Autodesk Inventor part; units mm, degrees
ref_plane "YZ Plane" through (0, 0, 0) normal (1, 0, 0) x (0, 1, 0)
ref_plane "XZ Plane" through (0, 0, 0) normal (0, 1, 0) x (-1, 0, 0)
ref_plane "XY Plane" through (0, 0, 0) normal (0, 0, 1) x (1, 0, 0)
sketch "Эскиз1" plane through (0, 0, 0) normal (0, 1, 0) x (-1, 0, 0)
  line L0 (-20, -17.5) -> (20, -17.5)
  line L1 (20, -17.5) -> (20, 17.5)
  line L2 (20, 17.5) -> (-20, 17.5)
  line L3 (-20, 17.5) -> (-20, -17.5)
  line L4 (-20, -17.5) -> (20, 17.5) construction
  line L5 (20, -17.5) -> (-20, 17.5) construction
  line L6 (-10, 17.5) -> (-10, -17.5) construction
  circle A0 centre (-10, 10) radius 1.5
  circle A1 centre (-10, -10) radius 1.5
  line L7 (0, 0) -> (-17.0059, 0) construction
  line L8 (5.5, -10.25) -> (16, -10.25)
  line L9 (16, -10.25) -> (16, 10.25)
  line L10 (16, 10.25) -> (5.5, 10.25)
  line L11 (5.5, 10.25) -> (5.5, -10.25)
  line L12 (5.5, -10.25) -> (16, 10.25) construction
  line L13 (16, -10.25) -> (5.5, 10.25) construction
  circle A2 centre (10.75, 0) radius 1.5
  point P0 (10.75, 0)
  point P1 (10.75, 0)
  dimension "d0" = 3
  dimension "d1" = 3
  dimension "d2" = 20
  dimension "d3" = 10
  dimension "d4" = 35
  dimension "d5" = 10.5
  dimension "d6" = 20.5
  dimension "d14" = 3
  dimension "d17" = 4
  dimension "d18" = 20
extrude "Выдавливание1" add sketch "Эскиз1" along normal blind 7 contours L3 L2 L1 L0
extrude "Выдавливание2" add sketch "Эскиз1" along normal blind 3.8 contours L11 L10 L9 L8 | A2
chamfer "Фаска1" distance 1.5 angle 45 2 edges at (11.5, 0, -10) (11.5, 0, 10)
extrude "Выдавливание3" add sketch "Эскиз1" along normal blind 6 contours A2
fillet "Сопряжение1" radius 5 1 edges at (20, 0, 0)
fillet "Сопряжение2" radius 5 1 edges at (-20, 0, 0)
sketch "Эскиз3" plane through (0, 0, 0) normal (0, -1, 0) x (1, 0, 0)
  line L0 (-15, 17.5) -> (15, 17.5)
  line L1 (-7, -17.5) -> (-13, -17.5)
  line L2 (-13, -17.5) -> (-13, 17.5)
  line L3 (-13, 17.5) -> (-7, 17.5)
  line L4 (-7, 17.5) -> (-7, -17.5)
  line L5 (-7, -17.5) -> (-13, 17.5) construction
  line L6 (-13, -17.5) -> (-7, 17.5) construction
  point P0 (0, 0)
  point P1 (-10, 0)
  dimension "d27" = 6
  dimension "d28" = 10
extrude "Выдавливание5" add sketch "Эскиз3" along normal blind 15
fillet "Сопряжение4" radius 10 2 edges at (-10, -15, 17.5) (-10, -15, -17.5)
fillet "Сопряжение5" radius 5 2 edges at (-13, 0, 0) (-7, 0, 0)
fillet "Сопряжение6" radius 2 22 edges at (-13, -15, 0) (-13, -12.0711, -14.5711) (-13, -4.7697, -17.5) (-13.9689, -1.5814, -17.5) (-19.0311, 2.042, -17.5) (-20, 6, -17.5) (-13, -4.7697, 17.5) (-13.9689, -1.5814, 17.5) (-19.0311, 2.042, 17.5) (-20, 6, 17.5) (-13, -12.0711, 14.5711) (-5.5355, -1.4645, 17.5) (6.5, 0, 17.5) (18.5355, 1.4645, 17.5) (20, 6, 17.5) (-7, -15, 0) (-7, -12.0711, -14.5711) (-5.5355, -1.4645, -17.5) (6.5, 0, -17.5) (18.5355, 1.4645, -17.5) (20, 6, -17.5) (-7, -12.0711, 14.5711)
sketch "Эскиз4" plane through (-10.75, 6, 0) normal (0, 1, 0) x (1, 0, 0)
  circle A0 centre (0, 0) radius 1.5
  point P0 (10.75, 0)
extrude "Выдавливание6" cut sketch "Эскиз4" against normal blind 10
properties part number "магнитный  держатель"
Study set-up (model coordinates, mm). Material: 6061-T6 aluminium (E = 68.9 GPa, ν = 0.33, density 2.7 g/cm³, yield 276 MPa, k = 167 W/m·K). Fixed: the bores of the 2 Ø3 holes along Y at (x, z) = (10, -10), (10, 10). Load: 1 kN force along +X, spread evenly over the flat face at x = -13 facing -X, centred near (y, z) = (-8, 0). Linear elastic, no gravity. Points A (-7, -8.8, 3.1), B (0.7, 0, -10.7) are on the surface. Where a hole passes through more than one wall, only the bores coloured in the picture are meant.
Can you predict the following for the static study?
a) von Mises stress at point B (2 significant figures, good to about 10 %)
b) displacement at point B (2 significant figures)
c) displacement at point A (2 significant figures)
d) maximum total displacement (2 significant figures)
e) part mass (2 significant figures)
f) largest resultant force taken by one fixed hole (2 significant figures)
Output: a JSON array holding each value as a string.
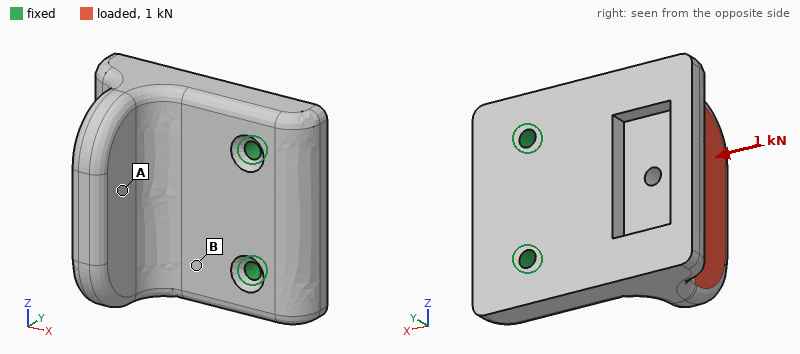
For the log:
["46 MPa", "0.017 mm", "0.066 mm", "0.10 mm", "31 g", "510 N"]
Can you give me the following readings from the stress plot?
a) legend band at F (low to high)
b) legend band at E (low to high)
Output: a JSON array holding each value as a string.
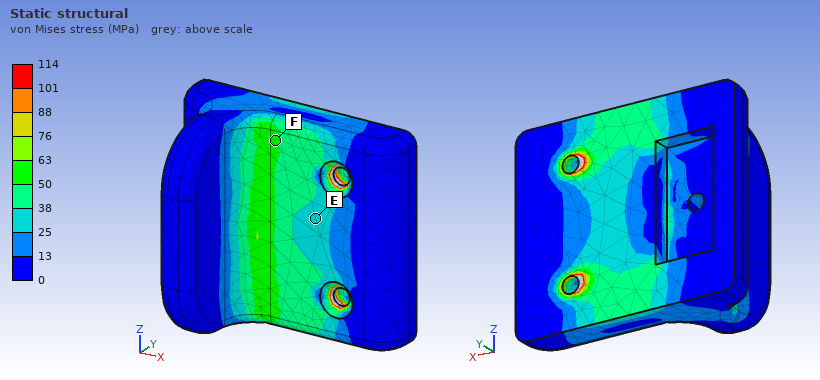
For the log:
["50 to 63 MPa", "25 to 38 MPa"]
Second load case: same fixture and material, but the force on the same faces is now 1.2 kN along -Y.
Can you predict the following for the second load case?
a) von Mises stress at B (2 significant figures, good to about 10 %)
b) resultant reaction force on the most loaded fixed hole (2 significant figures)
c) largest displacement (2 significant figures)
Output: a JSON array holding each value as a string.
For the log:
["57 MPa", "600 N", "0.16 mm"]
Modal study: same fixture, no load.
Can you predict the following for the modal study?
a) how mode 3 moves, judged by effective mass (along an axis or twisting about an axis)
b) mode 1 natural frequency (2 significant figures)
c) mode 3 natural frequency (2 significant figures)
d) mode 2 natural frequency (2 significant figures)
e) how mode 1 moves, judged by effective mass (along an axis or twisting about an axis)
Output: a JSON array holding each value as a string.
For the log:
["along Z", "4000 Hz", "13 kHz", "8300 Hz", "along Y"]
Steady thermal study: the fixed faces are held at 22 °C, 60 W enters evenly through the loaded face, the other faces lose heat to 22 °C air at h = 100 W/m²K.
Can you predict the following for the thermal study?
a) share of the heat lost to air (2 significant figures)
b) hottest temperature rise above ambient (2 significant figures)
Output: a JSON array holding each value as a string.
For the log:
["15 %", "46 K"]
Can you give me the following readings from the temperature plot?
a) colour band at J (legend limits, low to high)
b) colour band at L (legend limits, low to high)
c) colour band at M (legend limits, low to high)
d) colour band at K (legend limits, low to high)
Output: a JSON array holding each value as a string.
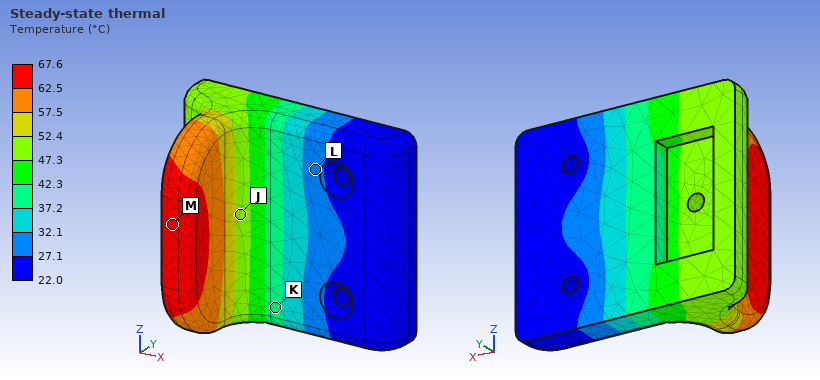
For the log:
["47.3 to 52.4 °C", "27.1 to 32.1 °C", "62.5 to 67.6 °C", "37.2 to 42.3 °C"]
